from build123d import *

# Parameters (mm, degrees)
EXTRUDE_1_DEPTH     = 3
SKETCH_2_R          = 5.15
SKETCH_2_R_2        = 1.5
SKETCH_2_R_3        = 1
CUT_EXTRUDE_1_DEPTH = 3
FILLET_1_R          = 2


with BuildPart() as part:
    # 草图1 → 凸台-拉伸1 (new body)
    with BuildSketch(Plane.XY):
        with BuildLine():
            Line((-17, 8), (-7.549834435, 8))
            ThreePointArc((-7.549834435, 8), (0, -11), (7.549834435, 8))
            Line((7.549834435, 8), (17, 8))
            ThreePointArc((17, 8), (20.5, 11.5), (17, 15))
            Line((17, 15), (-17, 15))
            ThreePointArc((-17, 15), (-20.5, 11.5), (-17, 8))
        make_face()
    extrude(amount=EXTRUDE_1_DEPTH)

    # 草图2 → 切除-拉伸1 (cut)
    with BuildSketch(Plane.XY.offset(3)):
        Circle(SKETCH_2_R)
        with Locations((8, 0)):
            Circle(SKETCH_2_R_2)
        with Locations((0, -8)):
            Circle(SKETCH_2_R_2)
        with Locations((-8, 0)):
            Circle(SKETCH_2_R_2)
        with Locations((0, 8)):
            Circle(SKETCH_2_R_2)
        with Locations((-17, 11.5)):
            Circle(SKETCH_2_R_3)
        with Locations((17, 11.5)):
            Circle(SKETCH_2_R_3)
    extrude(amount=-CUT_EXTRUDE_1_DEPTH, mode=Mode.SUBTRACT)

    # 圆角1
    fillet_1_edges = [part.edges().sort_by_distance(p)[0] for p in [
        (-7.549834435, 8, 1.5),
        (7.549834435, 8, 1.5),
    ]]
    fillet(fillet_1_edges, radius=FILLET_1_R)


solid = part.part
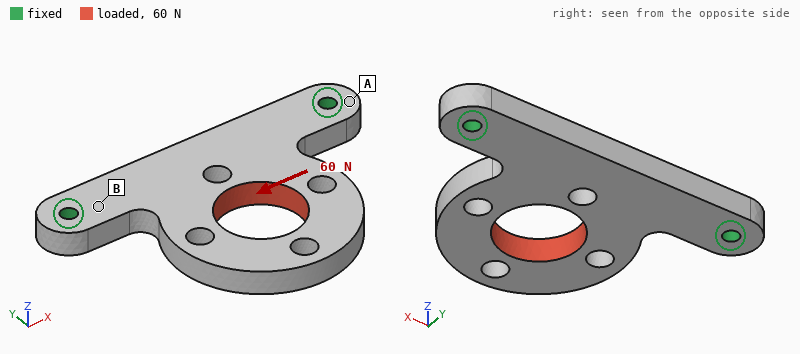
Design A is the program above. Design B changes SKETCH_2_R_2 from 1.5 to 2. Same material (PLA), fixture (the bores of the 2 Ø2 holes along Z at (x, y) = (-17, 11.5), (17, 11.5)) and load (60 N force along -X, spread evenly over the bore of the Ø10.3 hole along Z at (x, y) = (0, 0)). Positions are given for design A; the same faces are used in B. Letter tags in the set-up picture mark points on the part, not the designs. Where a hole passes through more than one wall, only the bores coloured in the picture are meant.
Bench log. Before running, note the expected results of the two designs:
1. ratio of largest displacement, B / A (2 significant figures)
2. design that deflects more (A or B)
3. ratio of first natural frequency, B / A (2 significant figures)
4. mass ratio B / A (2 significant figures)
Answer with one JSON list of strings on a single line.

["1.4", "B", "1.0", "0.96"]
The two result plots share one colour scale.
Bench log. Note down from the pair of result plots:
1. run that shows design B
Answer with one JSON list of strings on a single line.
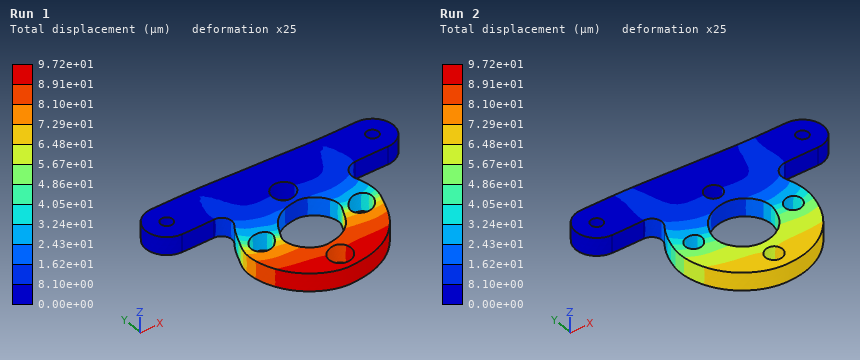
["Run 1"]
